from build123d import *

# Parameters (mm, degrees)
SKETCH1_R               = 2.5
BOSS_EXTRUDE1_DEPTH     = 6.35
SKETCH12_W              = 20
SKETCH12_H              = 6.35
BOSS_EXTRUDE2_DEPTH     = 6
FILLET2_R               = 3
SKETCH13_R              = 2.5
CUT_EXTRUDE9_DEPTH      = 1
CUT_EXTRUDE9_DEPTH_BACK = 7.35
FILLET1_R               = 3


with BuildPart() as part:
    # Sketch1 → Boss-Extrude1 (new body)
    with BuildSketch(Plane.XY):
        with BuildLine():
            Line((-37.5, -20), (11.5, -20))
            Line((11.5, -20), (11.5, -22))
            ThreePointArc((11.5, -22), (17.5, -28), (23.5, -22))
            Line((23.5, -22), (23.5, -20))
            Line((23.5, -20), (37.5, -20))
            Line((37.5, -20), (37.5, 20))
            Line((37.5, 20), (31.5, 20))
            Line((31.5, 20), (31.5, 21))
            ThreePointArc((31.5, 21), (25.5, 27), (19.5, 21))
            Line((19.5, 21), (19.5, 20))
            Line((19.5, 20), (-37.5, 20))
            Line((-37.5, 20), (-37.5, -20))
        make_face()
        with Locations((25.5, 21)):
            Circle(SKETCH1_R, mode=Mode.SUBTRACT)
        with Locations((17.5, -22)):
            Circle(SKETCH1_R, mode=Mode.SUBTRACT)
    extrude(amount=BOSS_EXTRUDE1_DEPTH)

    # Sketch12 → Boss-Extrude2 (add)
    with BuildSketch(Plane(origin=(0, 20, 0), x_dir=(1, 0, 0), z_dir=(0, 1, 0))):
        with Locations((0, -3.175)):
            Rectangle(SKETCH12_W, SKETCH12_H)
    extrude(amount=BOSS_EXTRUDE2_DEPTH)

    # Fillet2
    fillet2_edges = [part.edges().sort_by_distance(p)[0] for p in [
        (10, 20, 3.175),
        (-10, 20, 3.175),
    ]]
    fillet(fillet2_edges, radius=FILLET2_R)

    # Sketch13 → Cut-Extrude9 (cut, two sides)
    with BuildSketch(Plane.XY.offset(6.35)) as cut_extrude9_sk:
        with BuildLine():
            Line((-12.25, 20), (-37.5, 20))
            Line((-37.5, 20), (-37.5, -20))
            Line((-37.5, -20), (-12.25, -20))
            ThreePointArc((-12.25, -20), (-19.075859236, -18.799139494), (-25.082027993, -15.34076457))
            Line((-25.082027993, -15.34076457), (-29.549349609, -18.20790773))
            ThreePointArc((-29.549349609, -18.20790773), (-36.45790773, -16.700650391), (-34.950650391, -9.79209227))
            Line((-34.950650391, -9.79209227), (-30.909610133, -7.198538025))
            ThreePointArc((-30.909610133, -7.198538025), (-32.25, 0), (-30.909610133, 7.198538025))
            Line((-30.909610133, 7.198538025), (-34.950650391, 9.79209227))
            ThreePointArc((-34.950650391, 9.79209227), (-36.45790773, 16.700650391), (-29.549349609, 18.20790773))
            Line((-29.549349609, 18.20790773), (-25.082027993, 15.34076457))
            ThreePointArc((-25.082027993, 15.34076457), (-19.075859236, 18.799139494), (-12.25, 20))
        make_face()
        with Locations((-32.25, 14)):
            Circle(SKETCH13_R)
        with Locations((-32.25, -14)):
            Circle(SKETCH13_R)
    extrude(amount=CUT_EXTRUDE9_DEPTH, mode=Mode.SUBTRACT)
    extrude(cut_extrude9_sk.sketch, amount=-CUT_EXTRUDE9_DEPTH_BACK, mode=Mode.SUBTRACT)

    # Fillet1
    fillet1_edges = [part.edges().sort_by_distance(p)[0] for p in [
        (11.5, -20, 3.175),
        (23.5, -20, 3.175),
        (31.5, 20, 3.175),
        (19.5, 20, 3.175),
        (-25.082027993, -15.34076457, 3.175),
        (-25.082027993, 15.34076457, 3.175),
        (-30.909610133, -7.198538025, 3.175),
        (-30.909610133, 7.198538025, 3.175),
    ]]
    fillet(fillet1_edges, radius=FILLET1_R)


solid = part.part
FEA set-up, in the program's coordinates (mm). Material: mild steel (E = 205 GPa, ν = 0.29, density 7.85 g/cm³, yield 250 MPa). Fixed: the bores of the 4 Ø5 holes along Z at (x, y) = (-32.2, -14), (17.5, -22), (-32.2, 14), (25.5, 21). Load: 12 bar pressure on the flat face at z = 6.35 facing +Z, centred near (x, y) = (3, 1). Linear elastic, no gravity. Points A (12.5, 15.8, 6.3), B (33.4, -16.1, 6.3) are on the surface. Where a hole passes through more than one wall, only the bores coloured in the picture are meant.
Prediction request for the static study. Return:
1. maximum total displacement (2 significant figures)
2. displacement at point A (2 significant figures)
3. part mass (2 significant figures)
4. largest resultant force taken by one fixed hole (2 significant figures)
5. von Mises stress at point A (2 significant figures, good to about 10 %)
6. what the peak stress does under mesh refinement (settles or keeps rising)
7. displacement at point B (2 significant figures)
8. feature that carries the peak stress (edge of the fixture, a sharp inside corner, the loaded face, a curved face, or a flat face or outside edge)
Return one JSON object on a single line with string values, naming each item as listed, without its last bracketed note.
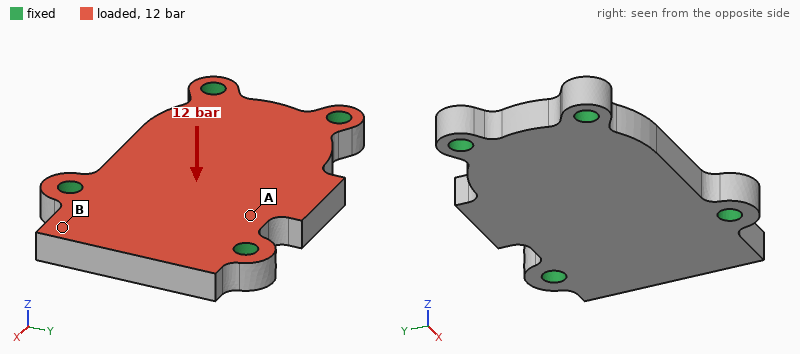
{"maximum total displacement": "14 µm", "displacement at point A": "7.1 µm", "part mass": "150 g", "largest resultant force taken by one fixed hole": "1.2 kN", "von Mises stress at point A": "26 MPa", "what the peak stress does under mesh refinement": "keeps rising", "displacement at point B": "3.4 µm", "feature that carries the peak stress": "edge of the fixture"}
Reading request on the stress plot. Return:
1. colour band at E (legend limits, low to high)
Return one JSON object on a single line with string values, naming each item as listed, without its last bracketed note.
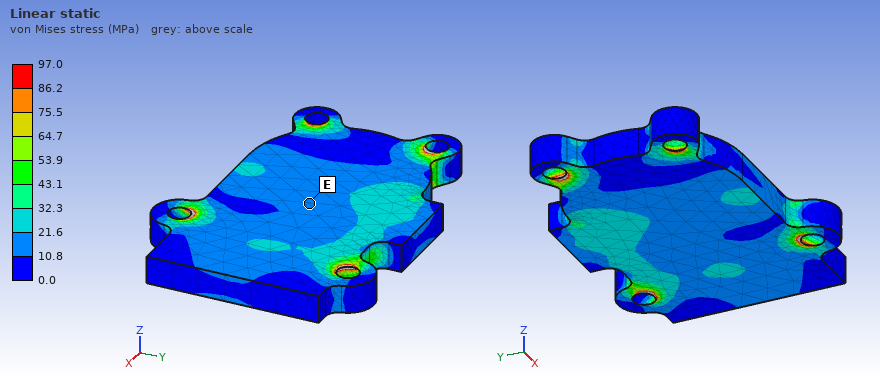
{"colour band at E": "10.8 to 21.6 MPa"}
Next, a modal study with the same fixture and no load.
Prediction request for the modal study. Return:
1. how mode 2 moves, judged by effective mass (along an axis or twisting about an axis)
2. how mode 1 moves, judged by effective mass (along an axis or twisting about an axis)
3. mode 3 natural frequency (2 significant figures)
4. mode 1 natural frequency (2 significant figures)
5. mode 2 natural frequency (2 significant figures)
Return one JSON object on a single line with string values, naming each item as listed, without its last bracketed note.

{"how mode 2 moves, judged by effective mass": "along Z", "how mode 1 moves, judged by effective mass": "along Z", "mode 3 natural frequency": "12 kHz", "mode 1 natural frequency": "8100 Hz", "mode 2 natural frequency": "11 kHz"}
